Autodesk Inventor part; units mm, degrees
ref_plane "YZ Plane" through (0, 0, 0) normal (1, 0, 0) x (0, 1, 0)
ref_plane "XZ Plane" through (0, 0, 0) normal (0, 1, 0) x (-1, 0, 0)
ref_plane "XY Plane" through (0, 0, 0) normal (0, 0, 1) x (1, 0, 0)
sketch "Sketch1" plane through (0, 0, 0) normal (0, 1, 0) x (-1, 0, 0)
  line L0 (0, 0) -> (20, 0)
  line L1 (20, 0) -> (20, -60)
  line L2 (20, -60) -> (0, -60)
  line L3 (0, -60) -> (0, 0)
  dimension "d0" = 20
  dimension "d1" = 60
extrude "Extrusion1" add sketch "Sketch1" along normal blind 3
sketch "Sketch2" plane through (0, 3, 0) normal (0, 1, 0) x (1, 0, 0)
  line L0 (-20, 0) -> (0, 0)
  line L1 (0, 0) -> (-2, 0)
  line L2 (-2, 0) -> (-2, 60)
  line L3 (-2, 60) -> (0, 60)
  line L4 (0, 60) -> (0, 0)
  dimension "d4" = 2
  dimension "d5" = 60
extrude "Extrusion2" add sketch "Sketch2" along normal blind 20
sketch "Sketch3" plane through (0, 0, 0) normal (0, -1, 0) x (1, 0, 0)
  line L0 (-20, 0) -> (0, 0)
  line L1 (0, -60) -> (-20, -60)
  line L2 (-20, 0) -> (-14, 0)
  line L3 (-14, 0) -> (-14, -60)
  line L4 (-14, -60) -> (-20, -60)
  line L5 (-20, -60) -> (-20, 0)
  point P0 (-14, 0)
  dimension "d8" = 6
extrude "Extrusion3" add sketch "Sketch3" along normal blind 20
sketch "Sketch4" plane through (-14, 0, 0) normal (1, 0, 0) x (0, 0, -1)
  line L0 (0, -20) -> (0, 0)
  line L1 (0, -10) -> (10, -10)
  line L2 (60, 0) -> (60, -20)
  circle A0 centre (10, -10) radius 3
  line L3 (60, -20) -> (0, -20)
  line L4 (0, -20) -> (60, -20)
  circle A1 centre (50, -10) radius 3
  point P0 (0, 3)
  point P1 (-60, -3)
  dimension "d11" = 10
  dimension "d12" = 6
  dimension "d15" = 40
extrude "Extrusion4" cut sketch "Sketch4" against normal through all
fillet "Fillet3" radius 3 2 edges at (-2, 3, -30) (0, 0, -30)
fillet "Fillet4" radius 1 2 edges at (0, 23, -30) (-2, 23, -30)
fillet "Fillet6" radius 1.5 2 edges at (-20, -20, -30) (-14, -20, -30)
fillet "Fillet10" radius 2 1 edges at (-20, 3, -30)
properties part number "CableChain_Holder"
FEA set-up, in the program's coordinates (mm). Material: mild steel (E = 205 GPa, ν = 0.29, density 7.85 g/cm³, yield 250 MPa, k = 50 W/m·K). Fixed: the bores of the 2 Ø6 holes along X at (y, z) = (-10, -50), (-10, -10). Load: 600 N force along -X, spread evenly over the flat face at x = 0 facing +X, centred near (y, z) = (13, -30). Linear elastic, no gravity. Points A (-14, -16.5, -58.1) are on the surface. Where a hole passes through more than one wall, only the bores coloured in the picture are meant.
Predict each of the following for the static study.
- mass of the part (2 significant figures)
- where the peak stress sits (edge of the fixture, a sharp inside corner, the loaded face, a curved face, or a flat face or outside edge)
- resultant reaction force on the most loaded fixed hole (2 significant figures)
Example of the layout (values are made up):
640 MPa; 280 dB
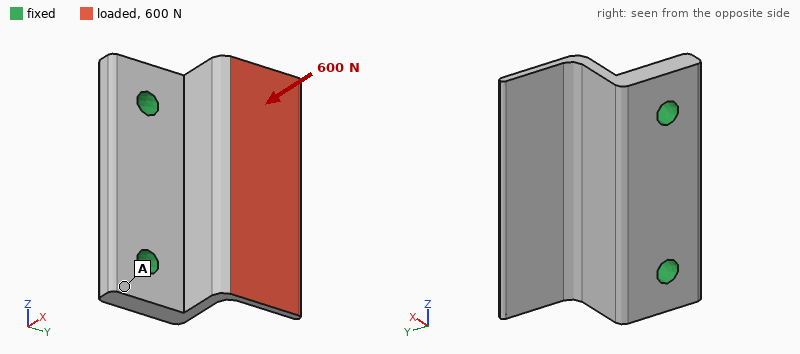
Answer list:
100 g; a curved face; 300 N
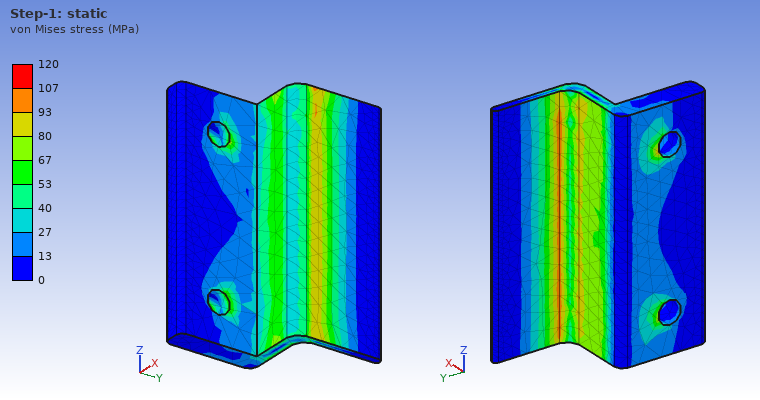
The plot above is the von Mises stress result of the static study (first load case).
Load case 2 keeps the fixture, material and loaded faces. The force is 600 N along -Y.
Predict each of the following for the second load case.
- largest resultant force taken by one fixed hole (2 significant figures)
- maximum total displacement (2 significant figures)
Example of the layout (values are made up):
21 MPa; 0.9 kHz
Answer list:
300 N; 79 µm
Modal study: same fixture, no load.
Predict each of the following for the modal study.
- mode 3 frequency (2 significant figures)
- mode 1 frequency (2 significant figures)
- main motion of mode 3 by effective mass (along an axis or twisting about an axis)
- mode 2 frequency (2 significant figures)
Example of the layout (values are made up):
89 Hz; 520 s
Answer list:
6900 Hz; 2700 Hz; along Y; 3900 Hz
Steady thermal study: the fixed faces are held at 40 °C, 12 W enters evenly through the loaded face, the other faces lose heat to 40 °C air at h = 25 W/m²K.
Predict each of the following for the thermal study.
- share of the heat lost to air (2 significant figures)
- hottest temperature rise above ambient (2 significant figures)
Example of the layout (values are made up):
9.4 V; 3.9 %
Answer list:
18 %; 40 K
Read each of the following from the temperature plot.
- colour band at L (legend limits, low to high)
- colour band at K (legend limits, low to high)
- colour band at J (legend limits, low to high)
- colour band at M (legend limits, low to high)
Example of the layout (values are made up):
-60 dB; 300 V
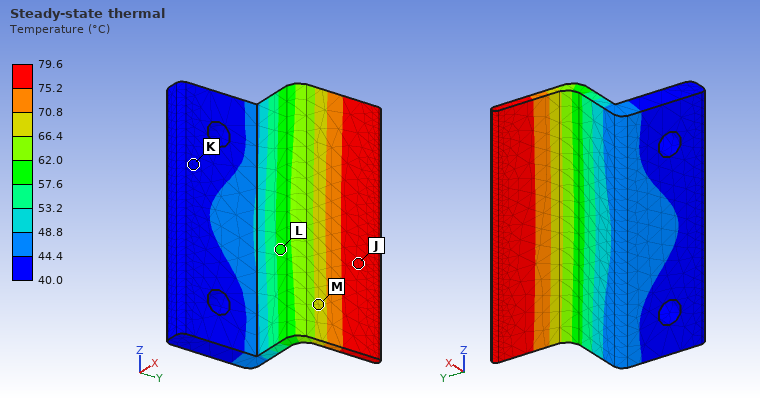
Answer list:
57.6 to 62.0 °C; 40.0 to 44.4 °C; 75.2 to 79.6 °C; 66.4 to 70.8 °C
